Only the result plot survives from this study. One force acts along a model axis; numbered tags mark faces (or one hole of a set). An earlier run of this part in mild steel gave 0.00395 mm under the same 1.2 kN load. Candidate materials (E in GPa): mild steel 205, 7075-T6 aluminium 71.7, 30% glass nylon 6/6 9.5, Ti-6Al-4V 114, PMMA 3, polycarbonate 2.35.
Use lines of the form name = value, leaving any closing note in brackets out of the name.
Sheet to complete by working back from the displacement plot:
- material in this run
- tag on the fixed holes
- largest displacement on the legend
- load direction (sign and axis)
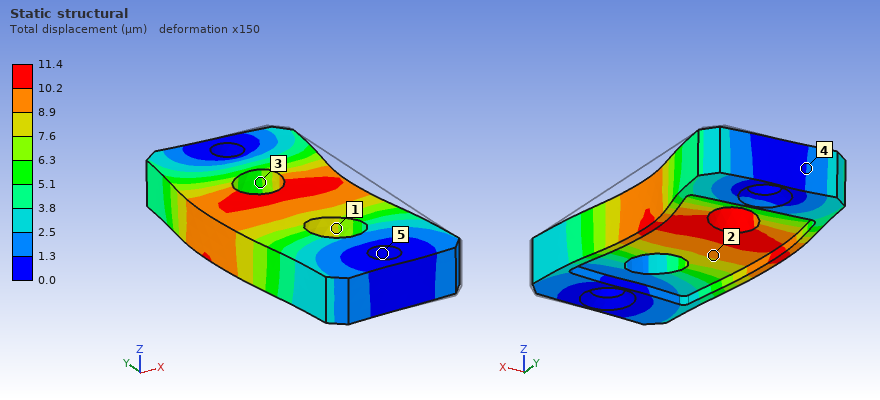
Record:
material in this run = 7075-T6 aluminium
tag on the fixed holes = 5
largest displacement on the legend = 11.4 µm
load direction = -X
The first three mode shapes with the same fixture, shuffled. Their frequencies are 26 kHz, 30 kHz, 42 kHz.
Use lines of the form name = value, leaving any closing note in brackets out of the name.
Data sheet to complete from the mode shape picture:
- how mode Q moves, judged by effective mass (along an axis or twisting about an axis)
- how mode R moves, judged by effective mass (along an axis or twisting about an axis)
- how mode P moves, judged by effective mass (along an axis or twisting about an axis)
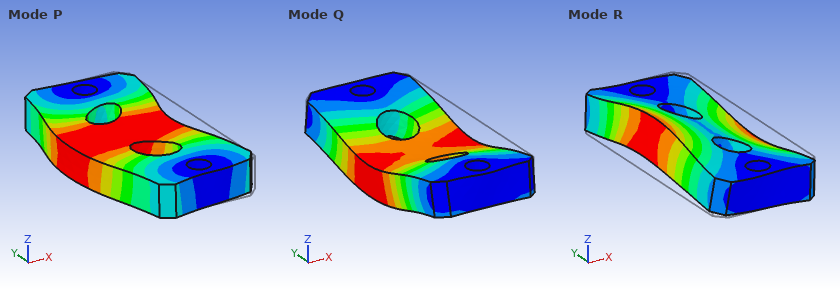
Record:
how mode Q moves, judged by effective mass = along Z
how mode R moves, judged by effective mass = twisting about Y
how mode P moves, judged by effective mass = along X
